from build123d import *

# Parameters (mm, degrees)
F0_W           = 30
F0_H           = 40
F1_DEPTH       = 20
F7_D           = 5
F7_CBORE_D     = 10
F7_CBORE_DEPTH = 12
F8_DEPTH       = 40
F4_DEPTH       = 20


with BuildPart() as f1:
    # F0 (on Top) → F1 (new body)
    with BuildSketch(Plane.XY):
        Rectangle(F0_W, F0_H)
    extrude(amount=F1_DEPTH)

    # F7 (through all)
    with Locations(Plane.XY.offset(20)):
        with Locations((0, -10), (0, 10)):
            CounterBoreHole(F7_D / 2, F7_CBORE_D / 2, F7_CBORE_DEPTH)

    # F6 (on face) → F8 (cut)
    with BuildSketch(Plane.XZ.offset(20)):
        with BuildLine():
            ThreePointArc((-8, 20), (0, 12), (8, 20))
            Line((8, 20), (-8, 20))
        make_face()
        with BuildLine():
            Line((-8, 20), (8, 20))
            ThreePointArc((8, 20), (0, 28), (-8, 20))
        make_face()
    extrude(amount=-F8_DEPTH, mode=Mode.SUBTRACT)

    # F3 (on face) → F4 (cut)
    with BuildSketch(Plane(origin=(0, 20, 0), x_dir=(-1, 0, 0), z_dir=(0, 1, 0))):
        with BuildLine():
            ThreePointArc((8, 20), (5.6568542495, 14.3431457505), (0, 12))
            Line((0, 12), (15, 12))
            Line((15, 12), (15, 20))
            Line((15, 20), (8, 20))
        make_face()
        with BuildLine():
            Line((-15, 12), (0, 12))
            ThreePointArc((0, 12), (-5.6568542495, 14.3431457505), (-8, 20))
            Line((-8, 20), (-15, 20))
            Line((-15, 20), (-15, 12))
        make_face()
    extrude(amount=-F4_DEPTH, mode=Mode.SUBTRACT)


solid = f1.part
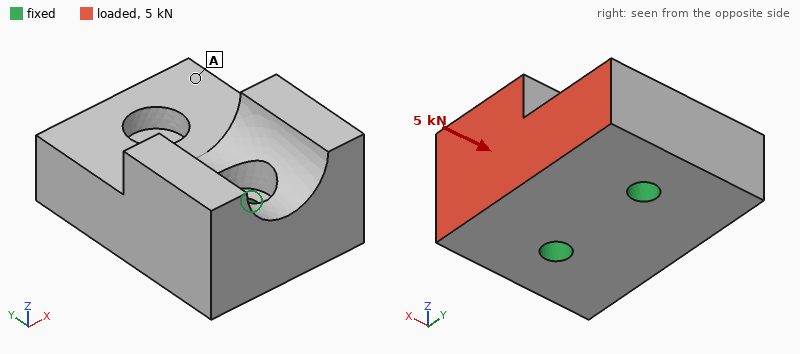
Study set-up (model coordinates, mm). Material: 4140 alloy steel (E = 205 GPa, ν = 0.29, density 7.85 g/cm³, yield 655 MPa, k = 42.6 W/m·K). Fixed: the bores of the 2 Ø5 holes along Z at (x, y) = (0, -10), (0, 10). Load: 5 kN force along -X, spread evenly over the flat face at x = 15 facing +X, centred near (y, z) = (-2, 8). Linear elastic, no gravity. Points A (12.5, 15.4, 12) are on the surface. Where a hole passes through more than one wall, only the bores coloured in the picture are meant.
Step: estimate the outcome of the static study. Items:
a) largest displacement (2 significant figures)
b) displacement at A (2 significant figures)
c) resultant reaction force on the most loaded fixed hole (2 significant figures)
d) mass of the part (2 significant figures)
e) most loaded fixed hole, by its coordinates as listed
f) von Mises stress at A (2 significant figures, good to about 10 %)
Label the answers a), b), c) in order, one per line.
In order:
a) 9.5 µm
b) 3.1 µm
c) 3.0 kN
d) 130 g
e) (0, -10)
f) 8.3 MPa
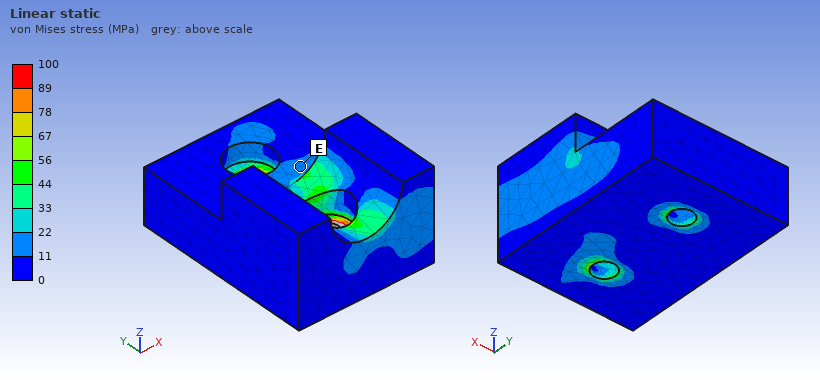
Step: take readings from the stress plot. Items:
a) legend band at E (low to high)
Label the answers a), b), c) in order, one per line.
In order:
a) 11 to 22 MPa
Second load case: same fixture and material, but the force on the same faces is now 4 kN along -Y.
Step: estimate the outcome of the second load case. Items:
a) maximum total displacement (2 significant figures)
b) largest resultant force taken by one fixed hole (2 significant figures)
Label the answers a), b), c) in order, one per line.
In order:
a) 5.9 µm
b) 3.3 kN
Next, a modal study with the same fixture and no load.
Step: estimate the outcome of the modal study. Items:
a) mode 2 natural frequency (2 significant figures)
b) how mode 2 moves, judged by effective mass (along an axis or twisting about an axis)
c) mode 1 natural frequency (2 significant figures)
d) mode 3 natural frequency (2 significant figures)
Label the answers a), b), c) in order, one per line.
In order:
a) 21 kHz
b) along Z
c) 13 kHz
d) 25 kHz
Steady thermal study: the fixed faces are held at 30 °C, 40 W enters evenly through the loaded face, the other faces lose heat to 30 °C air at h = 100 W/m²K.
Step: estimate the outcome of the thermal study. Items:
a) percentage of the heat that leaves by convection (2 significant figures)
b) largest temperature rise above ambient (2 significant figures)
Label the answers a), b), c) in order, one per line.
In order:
a) 12 %
b) 37 K
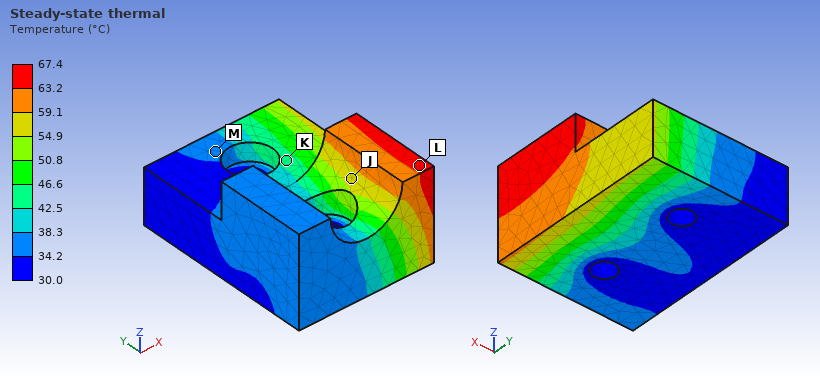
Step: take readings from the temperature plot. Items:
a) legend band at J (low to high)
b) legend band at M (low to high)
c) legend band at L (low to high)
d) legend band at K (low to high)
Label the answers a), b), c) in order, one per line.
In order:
a) 54.9 to 59.1 °C
b) 34.2 to 38.3 °C
c) 63.2 to 67.4 °C
d) 42.5 to 46.6 °C
